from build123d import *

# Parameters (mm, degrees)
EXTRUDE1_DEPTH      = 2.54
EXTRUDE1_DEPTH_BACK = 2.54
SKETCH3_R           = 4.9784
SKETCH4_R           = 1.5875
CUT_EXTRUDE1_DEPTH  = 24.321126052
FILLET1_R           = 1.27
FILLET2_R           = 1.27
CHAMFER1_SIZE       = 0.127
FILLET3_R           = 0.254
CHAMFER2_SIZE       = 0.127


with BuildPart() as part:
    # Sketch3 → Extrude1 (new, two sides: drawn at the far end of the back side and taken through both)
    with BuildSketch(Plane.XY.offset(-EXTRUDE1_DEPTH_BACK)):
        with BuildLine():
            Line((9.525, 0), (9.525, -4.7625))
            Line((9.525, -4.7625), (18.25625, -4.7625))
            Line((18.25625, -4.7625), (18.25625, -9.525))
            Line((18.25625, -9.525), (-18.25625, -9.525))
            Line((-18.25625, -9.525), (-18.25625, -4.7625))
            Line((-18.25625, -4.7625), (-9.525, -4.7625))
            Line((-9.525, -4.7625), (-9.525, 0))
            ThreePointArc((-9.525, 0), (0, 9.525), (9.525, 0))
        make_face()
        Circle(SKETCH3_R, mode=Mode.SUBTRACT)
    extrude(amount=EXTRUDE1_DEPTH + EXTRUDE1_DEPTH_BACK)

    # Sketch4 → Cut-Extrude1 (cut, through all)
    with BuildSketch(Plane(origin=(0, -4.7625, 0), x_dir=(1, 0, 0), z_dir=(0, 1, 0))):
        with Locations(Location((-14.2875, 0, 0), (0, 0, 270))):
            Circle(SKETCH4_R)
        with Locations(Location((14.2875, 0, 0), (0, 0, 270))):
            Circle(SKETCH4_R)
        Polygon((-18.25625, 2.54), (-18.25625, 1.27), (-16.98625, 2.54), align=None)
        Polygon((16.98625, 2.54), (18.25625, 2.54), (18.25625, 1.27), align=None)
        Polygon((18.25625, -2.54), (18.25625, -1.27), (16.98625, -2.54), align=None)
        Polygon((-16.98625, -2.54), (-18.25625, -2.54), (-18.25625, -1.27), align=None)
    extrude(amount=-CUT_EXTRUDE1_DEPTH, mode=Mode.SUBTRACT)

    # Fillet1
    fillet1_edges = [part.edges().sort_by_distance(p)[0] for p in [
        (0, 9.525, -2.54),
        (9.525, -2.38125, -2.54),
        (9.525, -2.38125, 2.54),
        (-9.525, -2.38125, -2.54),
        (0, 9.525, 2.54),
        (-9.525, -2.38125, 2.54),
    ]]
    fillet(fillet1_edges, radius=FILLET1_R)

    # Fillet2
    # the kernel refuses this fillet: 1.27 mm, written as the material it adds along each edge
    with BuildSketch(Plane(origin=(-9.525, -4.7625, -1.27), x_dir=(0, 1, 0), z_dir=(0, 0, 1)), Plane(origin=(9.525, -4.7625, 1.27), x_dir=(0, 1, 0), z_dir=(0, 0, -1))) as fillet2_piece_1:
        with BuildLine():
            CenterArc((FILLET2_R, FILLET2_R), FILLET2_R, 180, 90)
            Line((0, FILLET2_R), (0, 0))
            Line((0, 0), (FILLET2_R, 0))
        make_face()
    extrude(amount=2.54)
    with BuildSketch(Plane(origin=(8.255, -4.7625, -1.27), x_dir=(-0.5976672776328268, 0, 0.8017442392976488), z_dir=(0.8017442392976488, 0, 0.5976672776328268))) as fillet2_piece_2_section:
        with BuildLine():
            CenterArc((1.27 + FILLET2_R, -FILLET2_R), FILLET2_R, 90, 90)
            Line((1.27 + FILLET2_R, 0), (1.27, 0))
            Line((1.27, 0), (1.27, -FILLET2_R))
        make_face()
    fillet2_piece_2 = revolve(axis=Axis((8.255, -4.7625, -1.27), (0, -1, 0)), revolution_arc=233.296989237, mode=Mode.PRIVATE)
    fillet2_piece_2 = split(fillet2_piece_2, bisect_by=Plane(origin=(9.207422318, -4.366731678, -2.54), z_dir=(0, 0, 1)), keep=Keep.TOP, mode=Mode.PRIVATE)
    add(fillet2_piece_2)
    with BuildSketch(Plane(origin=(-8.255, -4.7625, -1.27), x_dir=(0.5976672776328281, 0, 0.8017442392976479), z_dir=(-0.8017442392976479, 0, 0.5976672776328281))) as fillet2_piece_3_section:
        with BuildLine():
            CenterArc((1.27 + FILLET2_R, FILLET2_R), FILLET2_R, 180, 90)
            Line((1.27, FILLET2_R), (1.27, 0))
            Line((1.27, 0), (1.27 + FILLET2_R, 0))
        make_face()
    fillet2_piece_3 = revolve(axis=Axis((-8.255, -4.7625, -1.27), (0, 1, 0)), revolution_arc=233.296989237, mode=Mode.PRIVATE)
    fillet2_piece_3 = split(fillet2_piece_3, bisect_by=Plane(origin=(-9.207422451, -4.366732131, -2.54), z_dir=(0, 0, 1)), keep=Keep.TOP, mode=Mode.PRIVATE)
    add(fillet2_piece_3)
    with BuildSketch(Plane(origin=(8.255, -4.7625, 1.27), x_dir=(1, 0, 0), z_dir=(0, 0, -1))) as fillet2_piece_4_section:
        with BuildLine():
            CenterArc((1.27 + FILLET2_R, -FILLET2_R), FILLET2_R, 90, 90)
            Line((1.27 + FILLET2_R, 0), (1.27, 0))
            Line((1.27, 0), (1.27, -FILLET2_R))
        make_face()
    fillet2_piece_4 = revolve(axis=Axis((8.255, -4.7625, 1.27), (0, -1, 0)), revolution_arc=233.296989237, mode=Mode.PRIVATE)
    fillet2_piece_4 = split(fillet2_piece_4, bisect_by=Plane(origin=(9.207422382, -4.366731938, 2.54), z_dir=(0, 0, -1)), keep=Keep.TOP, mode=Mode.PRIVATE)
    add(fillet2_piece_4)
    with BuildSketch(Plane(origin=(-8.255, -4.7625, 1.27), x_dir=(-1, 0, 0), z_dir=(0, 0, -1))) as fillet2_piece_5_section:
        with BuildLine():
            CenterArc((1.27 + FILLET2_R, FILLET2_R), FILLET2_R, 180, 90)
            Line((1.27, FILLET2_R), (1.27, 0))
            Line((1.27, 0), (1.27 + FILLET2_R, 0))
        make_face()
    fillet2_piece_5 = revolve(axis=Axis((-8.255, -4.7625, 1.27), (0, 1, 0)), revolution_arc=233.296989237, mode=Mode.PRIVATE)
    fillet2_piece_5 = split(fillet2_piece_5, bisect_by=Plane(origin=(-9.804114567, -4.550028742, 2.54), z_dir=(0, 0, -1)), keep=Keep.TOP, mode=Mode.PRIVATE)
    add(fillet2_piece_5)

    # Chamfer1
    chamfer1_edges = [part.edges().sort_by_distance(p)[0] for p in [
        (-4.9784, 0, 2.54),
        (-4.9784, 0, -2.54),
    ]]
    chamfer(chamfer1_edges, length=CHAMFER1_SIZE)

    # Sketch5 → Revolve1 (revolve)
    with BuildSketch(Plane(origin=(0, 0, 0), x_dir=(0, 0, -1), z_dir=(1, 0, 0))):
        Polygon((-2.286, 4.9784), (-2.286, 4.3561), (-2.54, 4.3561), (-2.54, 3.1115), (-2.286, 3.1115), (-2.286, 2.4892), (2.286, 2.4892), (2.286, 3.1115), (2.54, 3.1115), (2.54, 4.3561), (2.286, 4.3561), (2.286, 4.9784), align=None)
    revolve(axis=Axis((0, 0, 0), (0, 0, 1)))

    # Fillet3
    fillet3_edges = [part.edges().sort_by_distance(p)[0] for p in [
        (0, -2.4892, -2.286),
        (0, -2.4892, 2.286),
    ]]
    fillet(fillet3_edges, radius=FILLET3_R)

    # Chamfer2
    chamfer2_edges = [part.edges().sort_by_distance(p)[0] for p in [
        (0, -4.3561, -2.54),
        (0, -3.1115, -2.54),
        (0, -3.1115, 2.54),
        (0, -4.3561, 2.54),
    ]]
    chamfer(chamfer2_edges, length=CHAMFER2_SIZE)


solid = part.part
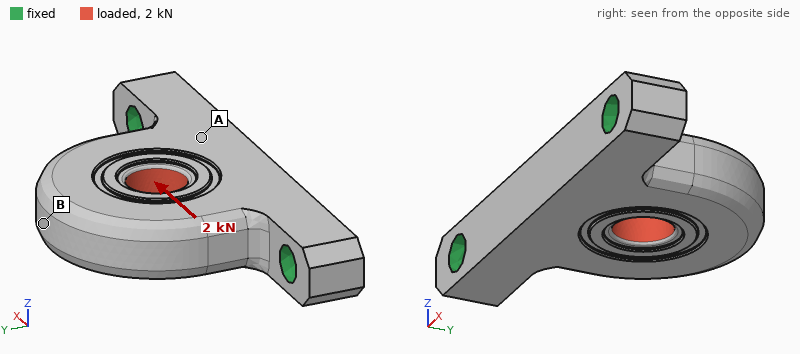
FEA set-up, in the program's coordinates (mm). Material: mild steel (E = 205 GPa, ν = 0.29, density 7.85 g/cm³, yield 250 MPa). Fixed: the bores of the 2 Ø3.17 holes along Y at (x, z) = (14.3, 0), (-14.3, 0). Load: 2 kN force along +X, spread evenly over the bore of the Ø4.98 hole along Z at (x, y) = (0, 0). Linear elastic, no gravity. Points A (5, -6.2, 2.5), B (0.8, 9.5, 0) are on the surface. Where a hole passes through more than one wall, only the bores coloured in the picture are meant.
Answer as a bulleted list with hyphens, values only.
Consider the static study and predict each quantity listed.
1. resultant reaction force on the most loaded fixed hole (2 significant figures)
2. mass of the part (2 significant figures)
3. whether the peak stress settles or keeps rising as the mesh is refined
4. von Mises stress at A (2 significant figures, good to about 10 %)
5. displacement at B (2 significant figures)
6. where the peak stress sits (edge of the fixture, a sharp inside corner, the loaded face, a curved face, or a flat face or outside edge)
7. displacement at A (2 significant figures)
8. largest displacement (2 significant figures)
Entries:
- 1.2 kN
- 14 g
- keeps rising
- 23 MPa
- 6.4 µm
- a sharp inside corner
- 1.6 µm
- 6.5 µm
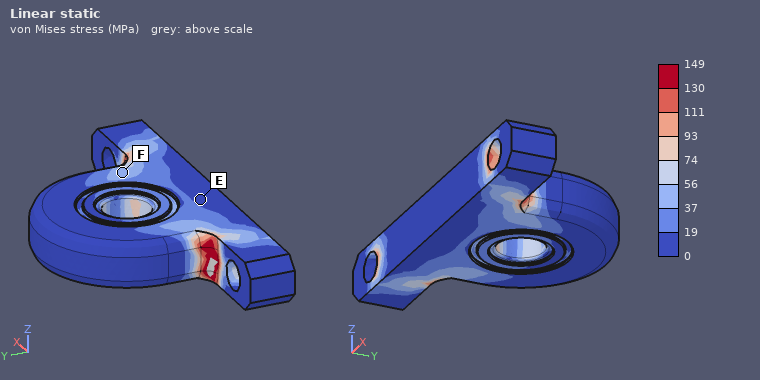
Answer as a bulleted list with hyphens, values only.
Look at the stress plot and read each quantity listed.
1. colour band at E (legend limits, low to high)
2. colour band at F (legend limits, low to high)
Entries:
- 0 to 19 MPa
- 37 to 56 MPa
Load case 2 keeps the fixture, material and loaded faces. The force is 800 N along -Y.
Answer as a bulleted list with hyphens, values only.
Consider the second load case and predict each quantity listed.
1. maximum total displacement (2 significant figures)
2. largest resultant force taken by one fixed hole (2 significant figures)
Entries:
- 2.8 µm
- 450 N
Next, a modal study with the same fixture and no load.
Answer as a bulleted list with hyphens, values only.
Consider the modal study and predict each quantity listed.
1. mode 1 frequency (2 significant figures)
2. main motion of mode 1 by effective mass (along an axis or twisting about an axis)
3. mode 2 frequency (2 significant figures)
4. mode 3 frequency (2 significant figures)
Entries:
- 8000 Hz
- along Z
- 28 kHz
- 28 kHz
